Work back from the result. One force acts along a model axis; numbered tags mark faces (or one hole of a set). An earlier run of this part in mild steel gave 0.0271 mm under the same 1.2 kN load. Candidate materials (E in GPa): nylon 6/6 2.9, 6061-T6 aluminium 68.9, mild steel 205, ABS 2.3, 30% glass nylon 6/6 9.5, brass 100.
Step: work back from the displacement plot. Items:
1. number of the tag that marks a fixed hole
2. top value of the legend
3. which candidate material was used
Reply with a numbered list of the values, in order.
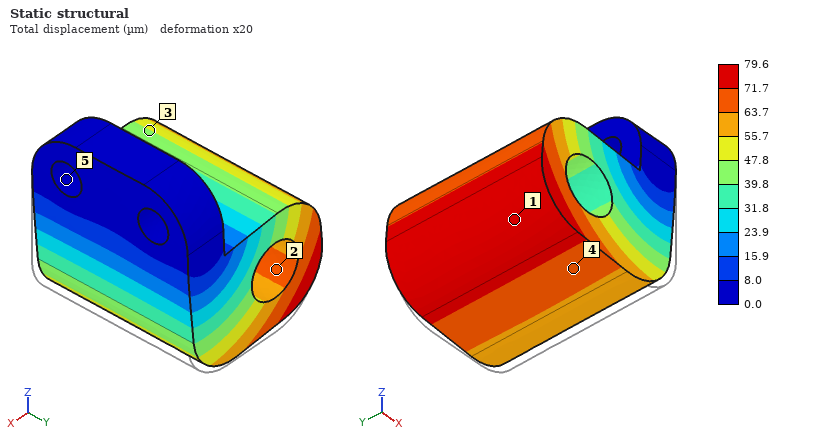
1. 5
2. 79.6 µm
3. 6061-T6 aluminium
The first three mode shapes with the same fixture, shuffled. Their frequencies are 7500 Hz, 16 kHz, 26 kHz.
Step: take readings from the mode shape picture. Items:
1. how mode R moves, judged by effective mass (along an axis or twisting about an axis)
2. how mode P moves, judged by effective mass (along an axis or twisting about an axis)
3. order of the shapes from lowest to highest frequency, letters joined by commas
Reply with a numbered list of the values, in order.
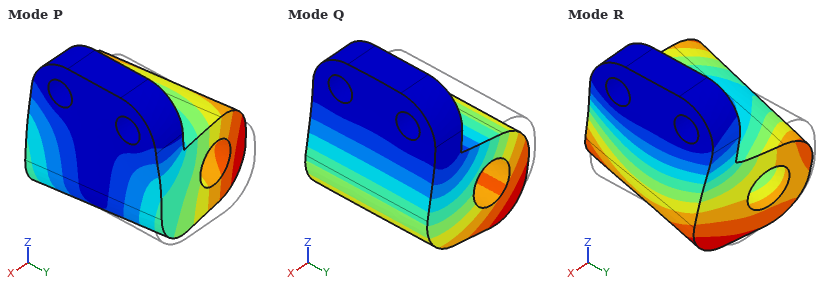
1. along Y
2. along Y
3. Q, P, R
